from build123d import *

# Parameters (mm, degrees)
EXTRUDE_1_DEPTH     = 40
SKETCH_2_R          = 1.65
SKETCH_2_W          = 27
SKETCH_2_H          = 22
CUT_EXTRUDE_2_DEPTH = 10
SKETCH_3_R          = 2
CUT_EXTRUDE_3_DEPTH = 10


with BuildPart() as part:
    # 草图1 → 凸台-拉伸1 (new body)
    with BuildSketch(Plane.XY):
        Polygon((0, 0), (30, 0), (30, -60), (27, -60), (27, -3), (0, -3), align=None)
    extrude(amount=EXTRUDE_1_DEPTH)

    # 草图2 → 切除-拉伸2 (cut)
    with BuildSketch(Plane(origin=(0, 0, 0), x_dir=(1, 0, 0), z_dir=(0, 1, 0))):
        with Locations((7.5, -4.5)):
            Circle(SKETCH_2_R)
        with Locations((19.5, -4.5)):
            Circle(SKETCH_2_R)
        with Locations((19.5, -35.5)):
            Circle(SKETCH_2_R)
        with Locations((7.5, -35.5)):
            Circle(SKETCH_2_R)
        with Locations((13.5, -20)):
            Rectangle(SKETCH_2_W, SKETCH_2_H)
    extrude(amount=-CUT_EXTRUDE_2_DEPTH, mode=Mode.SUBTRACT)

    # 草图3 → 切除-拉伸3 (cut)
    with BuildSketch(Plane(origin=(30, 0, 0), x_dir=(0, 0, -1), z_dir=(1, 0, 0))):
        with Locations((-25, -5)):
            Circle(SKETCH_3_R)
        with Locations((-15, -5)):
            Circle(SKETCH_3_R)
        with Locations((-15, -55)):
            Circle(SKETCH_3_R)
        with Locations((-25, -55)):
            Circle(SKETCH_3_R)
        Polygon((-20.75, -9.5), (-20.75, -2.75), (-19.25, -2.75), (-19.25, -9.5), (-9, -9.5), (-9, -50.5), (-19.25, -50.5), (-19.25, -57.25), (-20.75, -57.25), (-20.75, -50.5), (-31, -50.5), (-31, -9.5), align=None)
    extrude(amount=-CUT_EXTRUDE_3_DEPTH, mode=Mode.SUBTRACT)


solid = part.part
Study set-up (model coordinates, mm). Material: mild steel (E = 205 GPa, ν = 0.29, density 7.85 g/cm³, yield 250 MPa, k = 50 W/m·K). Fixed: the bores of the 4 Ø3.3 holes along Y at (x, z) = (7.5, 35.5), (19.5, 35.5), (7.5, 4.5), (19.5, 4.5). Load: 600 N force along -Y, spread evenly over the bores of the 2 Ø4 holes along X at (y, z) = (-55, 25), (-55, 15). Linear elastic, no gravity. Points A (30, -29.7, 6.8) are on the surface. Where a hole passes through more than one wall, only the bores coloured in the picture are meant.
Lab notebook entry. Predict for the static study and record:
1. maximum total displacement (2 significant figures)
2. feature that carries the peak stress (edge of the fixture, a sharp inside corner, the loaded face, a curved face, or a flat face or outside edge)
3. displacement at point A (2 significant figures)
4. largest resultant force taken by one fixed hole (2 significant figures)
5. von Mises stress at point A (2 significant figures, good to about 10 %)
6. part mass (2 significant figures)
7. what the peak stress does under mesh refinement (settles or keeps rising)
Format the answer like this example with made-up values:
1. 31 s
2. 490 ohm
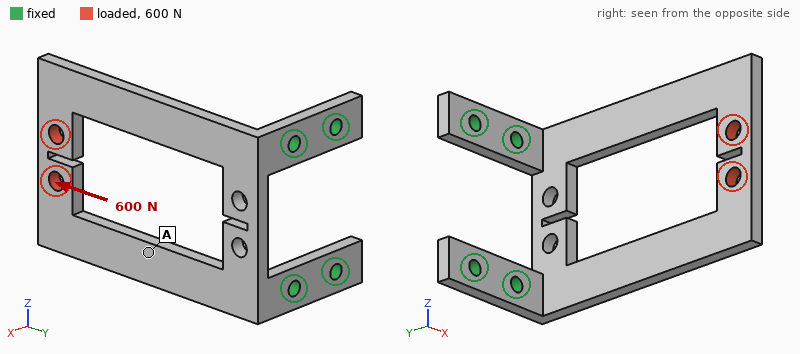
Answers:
1. 0.15 mm
2. edge of the fixture
3. 0.072 mm
4. 320 N
5. 25 MPa
6. 44 g
7. keeps rising
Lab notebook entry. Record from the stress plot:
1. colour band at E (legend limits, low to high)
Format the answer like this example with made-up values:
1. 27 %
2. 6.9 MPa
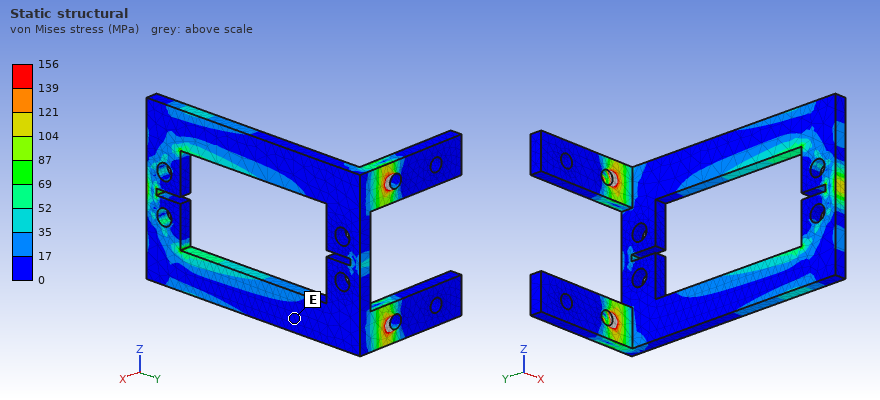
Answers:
1. 0 to 17 MPa
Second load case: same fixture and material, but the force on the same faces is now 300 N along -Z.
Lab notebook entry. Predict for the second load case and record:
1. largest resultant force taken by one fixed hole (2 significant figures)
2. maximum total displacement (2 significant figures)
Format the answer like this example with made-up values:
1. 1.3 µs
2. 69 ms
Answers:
1. 500 N
2. 0.14 mm
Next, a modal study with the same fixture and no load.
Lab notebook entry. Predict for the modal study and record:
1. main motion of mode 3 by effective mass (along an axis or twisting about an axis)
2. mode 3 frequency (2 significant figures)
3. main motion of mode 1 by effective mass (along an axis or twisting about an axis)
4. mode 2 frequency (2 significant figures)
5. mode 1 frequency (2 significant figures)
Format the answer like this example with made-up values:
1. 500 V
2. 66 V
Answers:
1. along Z
2. 2100 Hz
3. along X
4. 1500 Hz
5. 500 Hz
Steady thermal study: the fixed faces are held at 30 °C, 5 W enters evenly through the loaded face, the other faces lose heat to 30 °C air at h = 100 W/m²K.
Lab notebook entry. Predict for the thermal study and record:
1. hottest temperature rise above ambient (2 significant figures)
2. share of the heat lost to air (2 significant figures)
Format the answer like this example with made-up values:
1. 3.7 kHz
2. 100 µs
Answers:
1. 36 K
2. 92 %
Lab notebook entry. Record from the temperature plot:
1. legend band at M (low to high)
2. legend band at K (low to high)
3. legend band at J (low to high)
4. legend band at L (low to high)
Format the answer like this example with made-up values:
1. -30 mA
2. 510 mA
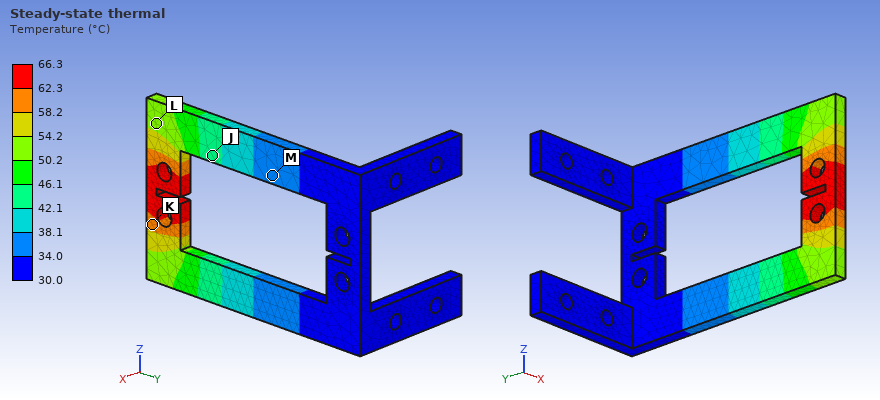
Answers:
1. 34.0 to 38.1 °C
2. 58.2 to 62.3 °C
3. 42.1 to 46.1 °C
4. 50.2 to 54.2 °C
